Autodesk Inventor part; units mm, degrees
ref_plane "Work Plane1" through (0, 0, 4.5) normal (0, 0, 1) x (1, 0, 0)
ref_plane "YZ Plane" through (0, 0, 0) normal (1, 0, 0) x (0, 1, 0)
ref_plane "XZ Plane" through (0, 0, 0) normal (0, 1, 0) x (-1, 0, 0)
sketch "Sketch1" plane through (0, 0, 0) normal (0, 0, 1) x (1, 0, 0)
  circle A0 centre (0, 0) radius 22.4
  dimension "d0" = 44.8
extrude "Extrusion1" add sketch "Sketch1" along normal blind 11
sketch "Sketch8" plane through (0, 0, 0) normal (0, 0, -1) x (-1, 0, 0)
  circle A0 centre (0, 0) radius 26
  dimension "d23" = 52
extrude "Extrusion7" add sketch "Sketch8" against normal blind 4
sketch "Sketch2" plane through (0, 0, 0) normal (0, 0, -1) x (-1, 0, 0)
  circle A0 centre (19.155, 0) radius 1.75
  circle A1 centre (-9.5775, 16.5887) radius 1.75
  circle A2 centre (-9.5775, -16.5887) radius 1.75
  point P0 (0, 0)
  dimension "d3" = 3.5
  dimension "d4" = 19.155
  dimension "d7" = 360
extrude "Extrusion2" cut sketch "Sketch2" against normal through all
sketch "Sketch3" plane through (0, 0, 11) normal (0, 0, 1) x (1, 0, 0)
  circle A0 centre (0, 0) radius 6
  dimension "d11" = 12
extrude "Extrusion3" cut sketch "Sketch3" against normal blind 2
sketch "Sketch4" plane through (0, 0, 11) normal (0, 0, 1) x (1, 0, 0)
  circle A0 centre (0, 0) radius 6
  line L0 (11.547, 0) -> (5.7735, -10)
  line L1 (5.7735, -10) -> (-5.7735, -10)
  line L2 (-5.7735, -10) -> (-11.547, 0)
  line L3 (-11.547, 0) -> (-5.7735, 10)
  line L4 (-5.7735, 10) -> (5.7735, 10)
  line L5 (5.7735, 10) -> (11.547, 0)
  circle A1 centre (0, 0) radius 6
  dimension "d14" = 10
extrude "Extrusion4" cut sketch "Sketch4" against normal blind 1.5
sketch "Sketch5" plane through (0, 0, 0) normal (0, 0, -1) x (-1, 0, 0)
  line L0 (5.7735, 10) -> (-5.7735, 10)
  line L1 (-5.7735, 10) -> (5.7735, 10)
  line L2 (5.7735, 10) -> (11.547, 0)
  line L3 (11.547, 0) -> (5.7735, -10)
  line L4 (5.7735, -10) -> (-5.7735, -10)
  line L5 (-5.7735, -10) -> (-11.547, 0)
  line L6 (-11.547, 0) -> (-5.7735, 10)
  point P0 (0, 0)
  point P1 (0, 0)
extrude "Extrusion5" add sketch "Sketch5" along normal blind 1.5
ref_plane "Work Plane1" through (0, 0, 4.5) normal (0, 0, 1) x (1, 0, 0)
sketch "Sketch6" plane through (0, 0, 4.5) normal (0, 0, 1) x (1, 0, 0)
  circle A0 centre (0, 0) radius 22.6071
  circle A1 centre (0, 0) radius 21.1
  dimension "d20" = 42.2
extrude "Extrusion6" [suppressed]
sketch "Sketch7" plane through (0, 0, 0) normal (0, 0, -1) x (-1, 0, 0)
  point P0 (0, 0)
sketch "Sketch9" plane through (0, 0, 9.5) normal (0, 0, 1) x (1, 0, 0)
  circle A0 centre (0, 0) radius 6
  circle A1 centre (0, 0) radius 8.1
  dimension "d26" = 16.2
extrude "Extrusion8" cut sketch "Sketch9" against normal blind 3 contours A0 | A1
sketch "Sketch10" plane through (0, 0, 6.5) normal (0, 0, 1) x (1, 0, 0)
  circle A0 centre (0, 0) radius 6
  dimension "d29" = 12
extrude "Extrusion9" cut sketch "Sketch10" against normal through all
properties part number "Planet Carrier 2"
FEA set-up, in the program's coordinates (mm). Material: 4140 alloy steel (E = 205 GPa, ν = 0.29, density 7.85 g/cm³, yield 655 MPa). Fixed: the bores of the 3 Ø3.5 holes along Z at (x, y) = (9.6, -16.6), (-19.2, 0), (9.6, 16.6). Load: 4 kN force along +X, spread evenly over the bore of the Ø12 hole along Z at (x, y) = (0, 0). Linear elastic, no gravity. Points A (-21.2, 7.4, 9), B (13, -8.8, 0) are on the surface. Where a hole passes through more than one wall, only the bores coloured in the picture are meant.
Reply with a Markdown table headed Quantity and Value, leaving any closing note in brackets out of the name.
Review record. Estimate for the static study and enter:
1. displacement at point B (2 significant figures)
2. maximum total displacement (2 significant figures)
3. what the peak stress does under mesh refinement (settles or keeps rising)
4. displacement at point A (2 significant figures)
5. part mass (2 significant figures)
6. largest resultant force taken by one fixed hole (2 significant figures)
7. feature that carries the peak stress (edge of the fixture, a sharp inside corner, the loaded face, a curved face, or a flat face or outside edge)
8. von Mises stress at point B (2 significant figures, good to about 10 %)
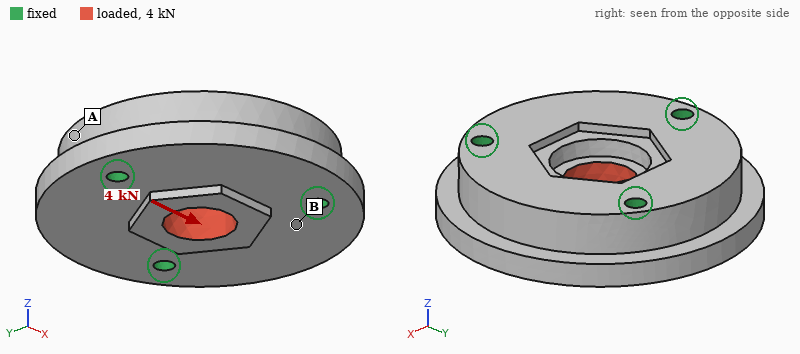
| Quantity | Value |
|---|---|
| displacement at point B | 0.89 µm |
| maximum total displacement | 1.9 µm |
| what the peak stress does under mesh refinement | keeps rising |
| displacement at point A | 0.36 µm |
| part mass | 140 g |
| largest resultant force taken by one fixed hole | 1.4 kN |
| feature that carries the peak stress | edge of the fixture |
| von Mises stress at point B | 11 MPa |
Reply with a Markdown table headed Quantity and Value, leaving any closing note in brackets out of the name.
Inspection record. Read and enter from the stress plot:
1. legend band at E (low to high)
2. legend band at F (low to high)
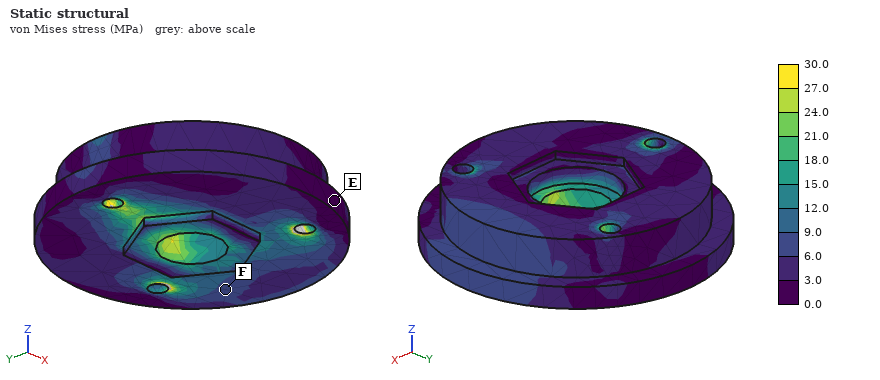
| Quantity | Value |
|---|---|
| legend band at E | 0.0 to 3.0 MPa |
| legend band at F | 6.0 to 9.0 MPa |
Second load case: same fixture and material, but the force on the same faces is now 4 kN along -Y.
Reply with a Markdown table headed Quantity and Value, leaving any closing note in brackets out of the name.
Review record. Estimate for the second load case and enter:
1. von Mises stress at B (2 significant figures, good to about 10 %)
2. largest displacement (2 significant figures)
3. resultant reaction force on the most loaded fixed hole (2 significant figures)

| Quantity | Value |
|---|---|
| von Mises stress at B | 6.1 MPa |
| largest displacement | 1.7 µm |
| resultant reaction force on the most loaded fixed hole | 1.4 kN |
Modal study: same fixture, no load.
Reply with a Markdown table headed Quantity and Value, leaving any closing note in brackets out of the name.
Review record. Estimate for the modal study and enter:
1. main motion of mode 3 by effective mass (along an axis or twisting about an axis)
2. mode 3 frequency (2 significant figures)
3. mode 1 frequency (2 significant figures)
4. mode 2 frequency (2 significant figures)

| Quantity | Value |
|---|---|
| main motion of mode 3 by effective mass | along Z |
| mode 3 frequency | 25 kHz |
| mode 1 frequency | 22 kHz |
| mode 2 frequency | 22 kHz |
